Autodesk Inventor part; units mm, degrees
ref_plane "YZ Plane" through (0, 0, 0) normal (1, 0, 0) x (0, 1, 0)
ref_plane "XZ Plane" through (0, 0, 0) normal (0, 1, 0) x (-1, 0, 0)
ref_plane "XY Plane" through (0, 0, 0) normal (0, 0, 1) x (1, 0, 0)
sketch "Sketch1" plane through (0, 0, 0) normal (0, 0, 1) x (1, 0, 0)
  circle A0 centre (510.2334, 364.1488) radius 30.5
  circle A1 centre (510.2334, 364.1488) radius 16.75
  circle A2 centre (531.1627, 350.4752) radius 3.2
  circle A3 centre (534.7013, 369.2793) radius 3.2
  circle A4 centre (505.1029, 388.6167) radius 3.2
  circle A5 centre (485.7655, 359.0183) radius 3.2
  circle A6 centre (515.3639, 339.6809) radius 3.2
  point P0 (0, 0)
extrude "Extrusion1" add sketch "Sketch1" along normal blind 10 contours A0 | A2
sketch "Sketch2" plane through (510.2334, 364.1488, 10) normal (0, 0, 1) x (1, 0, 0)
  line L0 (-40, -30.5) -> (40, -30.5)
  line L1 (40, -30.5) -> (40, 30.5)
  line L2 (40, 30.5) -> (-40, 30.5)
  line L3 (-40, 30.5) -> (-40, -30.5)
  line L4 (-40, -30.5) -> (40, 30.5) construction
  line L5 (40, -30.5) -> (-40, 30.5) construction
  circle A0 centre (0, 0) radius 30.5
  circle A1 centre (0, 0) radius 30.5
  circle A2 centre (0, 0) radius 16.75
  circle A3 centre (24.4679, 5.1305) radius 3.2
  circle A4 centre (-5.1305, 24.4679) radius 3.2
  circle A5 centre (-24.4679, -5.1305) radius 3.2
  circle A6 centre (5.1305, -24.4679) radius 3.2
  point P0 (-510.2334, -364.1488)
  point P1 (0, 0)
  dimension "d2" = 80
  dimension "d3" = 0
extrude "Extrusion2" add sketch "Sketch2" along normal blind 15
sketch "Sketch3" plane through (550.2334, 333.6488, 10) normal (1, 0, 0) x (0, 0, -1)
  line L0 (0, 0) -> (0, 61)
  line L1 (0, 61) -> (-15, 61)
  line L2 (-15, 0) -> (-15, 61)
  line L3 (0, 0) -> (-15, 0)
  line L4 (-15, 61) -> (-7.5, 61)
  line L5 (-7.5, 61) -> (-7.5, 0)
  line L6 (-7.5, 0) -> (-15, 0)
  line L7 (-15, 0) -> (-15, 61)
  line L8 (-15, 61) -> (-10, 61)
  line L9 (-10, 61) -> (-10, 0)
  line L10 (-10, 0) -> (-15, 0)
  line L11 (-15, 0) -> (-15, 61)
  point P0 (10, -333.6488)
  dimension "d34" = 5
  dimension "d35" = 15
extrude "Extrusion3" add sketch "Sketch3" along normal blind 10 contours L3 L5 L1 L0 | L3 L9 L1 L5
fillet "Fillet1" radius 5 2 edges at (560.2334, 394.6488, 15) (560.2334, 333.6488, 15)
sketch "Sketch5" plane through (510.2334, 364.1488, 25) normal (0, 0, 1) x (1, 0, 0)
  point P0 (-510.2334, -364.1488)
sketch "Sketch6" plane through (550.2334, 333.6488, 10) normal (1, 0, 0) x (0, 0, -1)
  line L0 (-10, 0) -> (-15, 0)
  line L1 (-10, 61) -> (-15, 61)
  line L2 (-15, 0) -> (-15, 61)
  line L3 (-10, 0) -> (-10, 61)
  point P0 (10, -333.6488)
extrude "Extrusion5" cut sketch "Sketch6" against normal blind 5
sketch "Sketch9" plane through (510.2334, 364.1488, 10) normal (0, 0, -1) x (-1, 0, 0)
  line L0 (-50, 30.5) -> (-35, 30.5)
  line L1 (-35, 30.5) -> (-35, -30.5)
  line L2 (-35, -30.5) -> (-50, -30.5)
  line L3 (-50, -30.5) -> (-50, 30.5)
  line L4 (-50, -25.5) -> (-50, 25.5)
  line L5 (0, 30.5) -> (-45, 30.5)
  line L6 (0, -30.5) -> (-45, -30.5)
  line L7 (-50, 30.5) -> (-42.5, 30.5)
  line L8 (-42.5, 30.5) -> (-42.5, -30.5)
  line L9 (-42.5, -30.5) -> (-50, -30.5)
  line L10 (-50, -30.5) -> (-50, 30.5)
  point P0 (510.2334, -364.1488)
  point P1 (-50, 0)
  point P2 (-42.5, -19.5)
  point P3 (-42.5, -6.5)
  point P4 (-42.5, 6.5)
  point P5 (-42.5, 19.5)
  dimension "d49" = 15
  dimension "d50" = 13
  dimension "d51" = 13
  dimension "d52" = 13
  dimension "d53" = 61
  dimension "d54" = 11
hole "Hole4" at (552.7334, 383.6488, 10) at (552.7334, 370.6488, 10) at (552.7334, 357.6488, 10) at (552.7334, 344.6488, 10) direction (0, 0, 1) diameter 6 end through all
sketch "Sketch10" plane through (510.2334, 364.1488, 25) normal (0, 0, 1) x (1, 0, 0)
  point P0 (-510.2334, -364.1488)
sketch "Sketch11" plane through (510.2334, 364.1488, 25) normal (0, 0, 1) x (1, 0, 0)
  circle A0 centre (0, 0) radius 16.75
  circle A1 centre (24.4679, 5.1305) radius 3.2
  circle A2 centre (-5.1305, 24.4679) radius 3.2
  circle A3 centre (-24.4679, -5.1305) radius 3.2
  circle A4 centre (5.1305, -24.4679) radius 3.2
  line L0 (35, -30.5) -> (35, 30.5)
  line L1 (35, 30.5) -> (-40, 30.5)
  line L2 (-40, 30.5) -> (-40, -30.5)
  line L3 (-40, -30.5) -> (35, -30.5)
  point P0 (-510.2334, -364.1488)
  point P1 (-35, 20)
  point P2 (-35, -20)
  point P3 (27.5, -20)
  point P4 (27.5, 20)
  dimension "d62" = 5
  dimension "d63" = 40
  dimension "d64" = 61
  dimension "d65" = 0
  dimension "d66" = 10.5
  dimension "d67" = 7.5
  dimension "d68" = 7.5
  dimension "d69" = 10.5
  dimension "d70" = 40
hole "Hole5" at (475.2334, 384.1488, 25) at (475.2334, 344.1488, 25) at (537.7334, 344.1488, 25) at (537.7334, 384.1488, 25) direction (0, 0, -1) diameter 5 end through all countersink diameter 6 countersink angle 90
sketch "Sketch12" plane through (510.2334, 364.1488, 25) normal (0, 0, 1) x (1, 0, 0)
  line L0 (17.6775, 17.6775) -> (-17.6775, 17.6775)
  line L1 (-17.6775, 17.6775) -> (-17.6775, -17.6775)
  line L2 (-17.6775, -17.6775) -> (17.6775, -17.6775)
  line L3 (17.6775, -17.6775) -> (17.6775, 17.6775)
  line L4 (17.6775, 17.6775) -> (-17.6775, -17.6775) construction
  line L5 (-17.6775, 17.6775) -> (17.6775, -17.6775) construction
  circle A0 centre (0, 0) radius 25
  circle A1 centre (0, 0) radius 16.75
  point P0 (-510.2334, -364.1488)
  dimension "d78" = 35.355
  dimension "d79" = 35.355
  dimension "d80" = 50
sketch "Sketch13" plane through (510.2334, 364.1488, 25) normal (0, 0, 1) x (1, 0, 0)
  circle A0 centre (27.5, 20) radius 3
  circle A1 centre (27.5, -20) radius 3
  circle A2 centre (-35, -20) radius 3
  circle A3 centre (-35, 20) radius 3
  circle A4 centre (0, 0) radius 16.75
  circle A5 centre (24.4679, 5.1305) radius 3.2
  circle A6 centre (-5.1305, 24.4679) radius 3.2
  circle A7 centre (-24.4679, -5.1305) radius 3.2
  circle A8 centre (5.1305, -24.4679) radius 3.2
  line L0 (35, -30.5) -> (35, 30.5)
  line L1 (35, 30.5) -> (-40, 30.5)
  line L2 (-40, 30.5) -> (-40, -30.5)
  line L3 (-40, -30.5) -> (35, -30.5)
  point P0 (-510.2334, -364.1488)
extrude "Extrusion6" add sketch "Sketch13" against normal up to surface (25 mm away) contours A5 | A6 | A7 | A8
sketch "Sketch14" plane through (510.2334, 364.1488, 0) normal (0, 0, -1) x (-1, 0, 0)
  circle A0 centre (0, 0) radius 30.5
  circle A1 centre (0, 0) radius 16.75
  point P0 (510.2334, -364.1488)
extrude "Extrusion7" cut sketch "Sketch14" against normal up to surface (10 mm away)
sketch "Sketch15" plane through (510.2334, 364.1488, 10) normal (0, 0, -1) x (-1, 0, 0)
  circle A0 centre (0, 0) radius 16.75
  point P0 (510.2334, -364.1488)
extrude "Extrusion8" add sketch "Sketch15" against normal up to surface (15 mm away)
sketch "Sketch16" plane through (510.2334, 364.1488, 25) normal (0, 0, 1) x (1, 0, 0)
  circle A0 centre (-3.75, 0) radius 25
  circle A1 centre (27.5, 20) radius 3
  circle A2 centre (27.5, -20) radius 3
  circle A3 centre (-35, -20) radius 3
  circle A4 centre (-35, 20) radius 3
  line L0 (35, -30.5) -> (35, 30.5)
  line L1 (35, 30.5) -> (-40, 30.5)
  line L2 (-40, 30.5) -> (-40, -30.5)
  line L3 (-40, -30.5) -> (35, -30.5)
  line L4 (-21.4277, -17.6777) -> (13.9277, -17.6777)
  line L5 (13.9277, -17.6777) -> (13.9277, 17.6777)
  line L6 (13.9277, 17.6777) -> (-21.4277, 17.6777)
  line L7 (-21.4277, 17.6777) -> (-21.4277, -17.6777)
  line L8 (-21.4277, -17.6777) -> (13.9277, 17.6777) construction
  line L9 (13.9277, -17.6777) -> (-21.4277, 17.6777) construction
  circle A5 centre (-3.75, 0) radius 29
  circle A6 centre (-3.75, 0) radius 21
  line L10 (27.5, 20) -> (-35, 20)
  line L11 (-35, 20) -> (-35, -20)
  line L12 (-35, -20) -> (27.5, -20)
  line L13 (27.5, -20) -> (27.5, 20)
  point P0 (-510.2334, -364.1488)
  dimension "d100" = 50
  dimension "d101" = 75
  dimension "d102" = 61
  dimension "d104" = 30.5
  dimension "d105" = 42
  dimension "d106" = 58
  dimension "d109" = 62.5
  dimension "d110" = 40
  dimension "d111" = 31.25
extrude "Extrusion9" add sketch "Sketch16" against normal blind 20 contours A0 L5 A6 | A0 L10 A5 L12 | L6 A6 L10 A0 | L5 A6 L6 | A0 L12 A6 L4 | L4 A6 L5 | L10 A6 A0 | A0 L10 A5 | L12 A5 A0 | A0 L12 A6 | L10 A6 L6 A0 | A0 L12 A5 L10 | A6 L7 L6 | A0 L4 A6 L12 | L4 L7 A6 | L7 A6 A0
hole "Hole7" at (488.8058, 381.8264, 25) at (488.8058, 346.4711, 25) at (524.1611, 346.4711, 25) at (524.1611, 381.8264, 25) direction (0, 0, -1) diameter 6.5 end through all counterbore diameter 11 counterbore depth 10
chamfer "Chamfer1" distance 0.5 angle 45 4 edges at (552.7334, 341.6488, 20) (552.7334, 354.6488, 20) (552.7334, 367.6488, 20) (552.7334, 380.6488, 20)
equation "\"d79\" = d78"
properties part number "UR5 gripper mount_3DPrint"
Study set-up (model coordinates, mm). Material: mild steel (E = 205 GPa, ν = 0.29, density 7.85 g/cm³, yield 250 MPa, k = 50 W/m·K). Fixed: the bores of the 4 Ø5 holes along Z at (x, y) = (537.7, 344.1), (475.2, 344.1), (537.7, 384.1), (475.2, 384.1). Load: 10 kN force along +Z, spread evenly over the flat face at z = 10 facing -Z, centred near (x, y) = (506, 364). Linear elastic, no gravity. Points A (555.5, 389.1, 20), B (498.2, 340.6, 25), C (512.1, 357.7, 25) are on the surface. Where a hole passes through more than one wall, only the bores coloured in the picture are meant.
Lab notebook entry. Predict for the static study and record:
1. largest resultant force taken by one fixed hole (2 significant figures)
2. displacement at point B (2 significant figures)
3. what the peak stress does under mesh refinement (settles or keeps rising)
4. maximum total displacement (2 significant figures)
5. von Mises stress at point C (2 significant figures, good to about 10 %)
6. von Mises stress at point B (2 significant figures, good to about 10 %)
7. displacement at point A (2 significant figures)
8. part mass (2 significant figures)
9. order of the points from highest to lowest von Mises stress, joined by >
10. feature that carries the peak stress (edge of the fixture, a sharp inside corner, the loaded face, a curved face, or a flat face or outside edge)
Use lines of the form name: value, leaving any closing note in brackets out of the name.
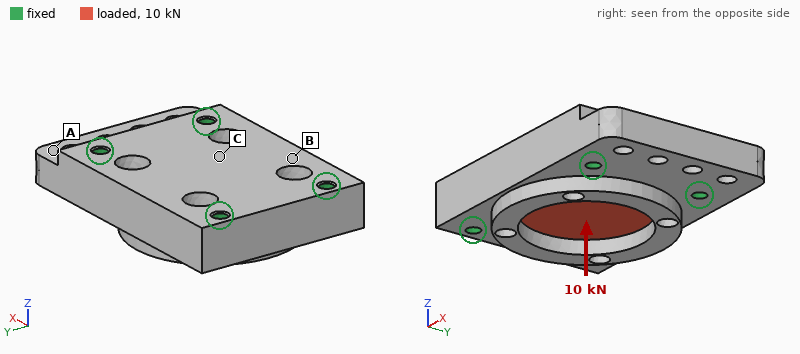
largest resultant force taken by one fixed hole: 2.5 kN
displacement at point B: 4.9 µm
what the peak stress does under mesh refinement: keeps rising
maximum total displacement: 7.5 µm
von Mises stress at point C: 23 MPa
von Mises stress at point B: 16 MPa
displacement at point A: 1.1 µm
part mass: 600 g
order of the points from highest to lowest von Mises stress, joined by >: C > B > A
feature that carries the peak stress: edge of the fixture
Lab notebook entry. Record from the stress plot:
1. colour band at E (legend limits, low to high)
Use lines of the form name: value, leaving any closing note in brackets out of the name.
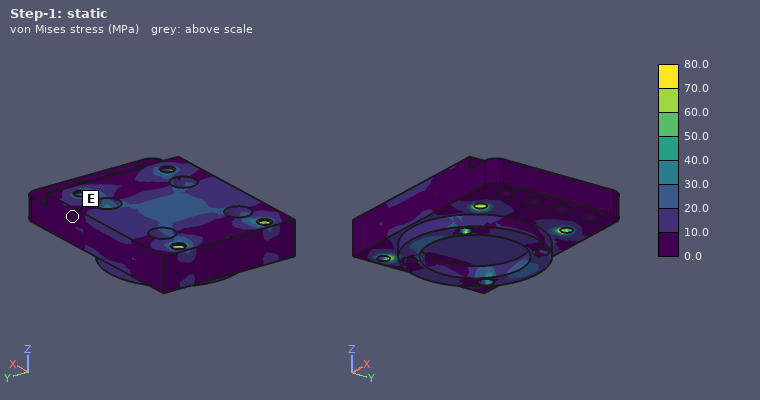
colour band at E: 0.0 to 10.0 MPa
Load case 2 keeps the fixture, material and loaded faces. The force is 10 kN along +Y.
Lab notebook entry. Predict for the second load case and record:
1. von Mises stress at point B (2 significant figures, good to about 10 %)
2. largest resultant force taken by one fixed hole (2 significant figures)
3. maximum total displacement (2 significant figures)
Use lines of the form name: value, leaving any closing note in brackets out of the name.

von Mises stress at point B: 5.5 MPa
largest resultant force taken by one fixed hole: 3.0 kN
maximum total displacement: 3.7 µm
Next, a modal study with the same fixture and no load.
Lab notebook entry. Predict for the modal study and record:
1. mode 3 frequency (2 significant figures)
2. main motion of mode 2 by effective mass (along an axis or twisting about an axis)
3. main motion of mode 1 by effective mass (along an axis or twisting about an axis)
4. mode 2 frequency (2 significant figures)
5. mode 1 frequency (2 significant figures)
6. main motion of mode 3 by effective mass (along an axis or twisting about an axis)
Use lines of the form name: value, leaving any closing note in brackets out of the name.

mode 3 frequency: 16 kHz
main motion of mode 2 by effective mass: twisting about X
main motion of mode 1 by effective mass: along Z
mode 2 frequency: 16 kHz
mode 1 frequency: 12 kHz
main motion of mode 3 by effective mass: along Z
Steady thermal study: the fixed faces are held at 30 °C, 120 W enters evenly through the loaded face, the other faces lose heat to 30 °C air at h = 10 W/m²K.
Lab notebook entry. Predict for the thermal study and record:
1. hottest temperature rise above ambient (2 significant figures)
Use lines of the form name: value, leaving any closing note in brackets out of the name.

hottest temperature rise above ambient: 53 K
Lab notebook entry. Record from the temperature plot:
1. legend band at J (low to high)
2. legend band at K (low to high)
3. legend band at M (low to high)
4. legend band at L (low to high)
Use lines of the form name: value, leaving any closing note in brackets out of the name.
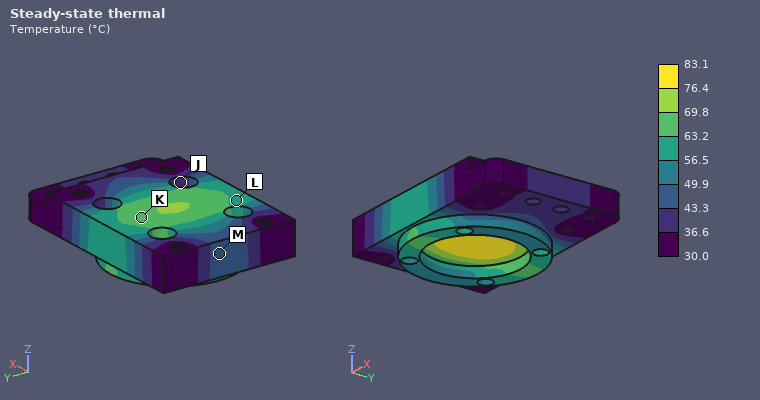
legend band at J: 36.6 to 43.3 °C
legend band at K: 63.2 to 69.8 °C
legend band at M: 43.3 to 49.9 °C
legend band at L: 56.5 to 63.2 °C
